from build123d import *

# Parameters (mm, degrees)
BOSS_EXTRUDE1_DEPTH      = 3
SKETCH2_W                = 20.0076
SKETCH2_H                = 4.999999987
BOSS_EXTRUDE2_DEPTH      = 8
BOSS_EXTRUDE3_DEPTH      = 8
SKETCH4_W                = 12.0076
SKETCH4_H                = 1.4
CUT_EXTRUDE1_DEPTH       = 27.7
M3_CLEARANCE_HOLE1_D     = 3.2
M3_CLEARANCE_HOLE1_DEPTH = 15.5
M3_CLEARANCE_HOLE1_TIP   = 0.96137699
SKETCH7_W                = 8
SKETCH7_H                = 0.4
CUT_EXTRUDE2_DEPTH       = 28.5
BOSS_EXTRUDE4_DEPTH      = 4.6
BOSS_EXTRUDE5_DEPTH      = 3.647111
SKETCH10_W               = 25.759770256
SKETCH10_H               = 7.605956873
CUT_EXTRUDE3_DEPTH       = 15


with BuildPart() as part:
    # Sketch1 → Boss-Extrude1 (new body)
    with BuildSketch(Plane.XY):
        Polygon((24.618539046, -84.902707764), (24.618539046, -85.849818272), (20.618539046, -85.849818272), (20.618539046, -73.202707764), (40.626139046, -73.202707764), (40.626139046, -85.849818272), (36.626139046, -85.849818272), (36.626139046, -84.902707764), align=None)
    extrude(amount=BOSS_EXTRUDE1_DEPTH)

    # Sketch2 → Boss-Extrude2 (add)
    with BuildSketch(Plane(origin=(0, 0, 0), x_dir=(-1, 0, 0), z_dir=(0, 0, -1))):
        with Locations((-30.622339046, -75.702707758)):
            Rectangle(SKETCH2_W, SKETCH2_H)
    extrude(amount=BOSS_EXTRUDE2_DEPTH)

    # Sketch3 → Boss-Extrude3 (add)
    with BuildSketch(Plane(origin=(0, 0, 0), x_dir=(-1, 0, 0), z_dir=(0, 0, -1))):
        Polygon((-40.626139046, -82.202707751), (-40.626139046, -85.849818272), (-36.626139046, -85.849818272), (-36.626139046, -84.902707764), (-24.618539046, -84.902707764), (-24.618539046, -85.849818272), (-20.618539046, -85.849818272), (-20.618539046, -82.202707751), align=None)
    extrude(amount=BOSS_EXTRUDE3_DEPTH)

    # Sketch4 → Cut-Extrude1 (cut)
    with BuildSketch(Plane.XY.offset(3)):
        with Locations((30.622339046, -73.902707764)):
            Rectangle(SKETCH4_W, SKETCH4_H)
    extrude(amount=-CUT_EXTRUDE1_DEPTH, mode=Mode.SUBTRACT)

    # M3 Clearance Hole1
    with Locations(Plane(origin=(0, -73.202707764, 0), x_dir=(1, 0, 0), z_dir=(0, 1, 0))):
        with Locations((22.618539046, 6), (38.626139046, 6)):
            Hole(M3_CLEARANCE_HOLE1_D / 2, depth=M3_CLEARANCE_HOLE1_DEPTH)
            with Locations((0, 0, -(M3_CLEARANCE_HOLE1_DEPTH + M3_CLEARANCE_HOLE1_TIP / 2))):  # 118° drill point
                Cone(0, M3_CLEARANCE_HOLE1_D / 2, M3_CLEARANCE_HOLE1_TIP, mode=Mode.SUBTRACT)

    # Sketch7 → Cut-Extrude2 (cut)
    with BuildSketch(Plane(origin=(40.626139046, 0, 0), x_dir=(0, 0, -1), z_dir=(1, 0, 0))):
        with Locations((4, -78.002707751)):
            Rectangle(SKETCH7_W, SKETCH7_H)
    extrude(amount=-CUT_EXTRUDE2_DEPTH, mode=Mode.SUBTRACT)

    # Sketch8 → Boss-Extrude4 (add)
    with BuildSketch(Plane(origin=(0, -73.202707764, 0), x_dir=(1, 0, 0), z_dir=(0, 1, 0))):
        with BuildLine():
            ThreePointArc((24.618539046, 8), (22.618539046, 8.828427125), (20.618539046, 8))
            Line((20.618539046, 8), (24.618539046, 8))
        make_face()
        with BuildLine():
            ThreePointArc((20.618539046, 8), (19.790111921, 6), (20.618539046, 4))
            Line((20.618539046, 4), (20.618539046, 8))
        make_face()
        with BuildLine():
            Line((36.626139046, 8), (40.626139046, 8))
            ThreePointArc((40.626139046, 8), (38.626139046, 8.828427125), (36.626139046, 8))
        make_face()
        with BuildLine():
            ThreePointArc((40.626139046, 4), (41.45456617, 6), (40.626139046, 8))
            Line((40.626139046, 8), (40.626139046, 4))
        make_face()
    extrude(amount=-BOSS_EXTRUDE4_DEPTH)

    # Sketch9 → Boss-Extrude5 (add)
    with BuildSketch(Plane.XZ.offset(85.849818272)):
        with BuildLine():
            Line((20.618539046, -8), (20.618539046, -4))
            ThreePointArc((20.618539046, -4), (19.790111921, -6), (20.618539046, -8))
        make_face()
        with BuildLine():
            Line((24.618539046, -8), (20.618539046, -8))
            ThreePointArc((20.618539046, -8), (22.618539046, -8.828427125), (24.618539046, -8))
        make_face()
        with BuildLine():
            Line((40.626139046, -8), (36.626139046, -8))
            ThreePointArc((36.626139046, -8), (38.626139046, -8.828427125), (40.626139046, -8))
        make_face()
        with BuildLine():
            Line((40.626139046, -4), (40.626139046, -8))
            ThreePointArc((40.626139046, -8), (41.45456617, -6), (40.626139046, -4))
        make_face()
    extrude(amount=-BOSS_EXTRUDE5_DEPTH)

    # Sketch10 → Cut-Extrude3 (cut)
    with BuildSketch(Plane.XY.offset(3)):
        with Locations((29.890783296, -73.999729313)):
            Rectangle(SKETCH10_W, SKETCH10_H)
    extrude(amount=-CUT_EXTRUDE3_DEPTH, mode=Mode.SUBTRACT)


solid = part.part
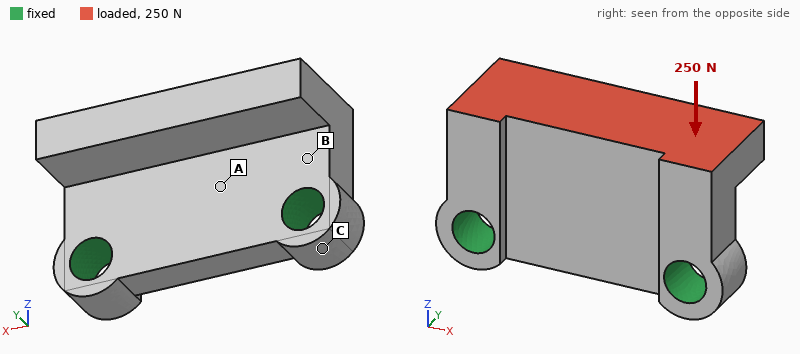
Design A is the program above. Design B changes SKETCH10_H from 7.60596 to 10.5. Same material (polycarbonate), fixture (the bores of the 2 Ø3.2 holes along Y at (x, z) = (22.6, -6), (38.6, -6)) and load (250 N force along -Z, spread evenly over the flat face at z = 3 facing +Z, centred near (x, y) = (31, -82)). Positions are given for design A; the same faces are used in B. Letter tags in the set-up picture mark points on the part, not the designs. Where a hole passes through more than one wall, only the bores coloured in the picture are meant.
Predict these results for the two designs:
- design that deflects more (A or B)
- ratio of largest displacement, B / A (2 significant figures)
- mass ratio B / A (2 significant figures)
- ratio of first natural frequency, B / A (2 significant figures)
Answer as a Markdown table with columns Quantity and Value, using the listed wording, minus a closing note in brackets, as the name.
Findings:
| Quantity | Value |
|---|---|
| design that deflects more | A |
| ratio of largest displacement, B / A | 0.61 |
| mass ratio B / A | 0.91 |
| ratio of first natural frequency, B / A | 1.2 |
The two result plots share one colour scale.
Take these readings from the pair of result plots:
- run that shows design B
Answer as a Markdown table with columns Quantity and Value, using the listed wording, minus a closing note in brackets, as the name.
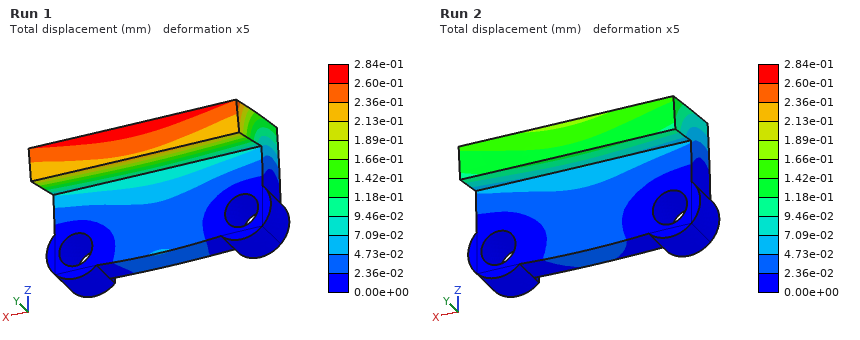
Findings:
| Quantity | Value |
|---|---|
| run that shows design B | Run 2 |
